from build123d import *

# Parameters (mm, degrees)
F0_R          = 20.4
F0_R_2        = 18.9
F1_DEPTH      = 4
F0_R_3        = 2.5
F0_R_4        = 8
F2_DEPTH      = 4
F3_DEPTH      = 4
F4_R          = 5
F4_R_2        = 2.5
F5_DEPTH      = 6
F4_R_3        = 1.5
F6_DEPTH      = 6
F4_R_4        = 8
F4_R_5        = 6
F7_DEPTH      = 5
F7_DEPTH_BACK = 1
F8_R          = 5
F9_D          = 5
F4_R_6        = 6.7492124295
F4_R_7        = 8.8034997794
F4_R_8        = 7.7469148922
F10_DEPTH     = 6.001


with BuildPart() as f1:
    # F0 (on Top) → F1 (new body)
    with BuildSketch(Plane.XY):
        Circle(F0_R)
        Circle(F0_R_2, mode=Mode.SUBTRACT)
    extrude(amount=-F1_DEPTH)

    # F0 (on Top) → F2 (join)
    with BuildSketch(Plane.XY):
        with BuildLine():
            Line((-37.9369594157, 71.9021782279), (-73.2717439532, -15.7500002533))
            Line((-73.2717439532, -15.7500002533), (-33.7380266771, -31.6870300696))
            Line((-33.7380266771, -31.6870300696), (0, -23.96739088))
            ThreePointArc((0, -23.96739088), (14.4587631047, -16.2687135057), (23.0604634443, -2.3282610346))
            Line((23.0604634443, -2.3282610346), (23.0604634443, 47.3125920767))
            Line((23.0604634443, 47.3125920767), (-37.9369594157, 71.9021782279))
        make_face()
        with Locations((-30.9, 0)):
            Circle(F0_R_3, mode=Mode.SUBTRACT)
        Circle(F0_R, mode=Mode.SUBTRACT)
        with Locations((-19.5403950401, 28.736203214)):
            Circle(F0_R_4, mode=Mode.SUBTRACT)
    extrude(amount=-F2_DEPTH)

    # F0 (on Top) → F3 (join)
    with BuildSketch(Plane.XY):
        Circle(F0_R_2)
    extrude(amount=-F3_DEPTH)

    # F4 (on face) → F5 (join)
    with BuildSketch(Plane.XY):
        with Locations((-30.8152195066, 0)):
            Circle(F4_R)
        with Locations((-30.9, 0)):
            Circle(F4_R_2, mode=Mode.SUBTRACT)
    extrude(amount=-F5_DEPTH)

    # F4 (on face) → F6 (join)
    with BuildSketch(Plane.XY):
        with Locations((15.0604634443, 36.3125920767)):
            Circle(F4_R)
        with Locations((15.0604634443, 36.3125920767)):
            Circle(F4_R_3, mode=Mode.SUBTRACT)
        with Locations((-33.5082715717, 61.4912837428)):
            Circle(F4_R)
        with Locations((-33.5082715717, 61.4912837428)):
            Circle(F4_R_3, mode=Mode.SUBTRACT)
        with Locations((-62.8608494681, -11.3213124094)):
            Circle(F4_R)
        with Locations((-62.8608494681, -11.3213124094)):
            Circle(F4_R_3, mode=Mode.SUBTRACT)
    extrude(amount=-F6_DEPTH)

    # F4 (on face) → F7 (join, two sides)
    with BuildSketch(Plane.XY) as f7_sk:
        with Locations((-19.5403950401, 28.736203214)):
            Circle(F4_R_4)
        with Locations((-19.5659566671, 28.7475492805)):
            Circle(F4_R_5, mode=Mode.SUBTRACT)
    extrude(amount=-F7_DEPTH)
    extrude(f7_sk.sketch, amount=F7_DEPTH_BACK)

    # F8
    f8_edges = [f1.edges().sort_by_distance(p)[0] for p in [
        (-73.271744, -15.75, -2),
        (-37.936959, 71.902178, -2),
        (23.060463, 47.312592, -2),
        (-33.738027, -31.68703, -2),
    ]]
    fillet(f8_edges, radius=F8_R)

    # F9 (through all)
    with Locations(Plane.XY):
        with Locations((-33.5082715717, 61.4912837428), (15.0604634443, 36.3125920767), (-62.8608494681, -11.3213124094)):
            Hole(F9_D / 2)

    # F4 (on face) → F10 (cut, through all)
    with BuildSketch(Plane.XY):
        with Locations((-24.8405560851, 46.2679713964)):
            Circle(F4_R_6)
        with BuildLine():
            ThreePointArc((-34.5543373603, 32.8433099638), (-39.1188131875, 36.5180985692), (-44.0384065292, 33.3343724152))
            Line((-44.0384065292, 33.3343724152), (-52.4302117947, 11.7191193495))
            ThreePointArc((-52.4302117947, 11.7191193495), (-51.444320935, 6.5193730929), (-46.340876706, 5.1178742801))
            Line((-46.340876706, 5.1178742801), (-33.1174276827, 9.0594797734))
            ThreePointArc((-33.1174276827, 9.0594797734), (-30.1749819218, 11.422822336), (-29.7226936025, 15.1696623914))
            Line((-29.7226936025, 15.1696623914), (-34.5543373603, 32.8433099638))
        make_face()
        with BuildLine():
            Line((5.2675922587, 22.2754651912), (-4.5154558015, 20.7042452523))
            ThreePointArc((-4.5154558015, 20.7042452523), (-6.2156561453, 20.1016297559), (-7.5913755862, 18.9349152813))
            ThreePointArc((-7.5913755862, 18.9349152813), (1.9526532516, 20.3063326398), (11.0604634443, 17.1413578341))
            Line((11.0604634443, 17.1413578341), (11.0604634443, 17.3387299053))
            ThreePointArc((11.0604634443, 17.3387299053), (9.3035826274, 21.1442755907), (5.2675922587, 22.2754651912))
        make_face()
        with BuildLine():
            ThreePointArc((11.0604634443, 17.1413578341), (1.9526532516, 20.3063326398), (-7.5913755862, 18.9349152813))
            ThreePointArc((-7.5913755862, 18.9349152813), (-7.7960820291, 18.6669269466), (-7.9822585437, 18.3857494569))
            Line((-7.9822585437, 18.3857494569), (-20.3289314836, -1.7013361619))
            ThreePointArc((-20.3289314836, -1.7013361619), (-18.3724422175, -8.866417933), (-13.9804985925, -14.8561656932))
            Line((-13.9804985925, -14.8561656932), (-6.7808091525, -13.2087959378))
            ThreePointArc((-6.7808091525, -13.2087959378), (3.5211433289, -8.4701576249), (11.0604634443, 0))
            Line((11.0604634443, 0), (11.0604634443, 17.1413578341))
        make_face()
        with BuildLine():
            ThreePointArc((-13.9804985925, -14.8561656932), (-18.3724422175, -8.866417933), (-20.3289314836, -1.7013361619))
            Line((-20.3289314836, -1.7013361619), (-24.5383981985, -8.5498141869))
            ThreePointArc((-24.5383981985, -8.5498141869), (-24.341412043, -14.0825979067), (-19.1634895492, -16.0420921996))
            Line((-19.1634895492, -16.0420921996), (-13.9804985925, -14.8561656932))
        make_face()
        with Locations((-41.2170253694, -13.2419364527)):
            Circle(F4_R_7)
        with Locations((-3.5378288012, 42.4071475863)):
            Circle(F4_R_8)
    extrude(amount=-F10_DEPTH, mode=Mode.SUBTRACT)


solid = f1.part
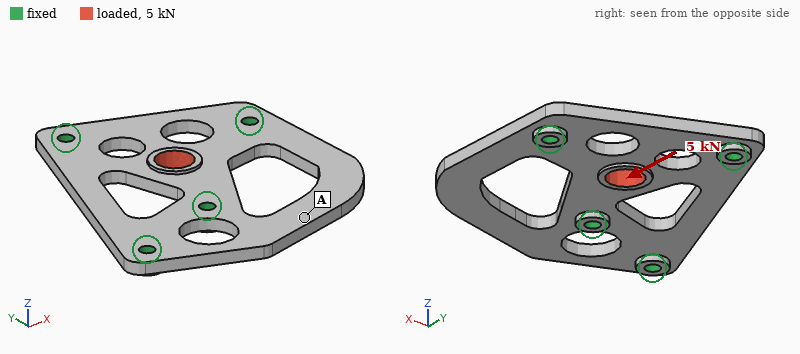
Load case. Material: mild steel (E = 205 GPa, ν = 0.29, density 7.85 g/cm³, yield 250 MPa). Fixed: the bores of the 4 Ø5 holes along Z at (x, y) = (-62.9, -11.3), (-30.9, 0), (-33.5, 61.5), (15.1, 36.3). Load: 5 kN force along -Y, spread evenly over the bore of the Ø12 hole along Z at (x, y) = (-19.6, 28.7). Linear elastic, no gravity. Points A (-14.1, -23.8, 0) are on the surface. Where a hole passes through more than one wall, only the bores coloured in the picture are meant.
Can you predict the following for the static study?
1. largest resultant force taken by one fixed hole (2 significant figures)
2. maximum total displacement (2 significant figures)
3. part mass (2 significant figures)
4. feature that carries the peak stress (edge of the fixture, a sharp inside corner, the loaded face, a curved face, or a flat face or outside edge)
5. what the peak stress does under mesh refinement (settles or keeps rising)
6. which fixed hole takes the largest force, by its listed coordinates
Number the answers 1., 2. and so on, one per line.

1. 2.4 kN
2. 9.6 µm
3. 150 g
4. edge of the fixture
5. keeps rising
6. (-30.9, 0)
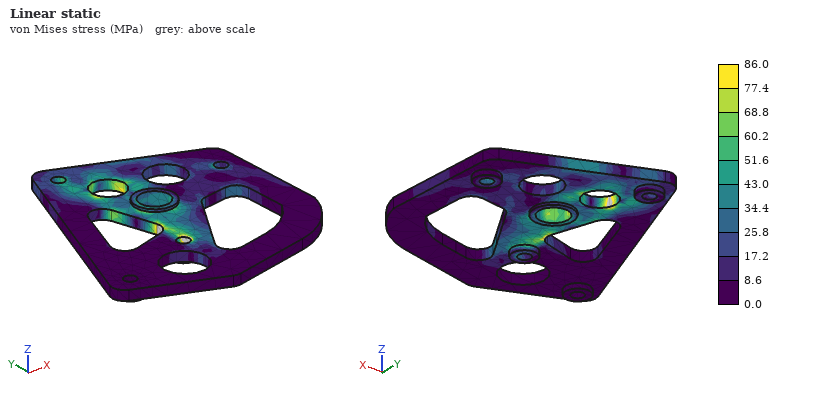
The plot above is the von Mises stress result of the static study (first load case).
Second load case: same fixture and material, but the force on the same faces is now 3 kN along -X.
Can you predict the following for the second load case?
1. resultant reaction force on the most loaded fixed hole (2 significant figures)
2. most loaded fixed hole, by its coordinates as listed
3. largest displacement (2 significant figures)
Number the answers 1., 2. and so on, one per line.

1. 1.6 kN
2. (15.1, 36.3)
3. 7.7 µm
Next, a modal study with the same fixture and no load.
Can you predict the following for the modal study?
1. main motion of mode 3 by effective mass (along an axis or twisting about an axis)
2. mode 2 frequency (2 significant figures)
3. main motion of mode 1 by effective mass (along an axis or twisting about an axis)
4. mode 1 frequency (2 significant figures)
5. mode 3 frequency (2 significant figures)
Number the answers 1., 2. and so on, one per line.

1. along Z
2. 4100 Hz
3. along Z
4. 1700 Hz
5. 4900 Hz
